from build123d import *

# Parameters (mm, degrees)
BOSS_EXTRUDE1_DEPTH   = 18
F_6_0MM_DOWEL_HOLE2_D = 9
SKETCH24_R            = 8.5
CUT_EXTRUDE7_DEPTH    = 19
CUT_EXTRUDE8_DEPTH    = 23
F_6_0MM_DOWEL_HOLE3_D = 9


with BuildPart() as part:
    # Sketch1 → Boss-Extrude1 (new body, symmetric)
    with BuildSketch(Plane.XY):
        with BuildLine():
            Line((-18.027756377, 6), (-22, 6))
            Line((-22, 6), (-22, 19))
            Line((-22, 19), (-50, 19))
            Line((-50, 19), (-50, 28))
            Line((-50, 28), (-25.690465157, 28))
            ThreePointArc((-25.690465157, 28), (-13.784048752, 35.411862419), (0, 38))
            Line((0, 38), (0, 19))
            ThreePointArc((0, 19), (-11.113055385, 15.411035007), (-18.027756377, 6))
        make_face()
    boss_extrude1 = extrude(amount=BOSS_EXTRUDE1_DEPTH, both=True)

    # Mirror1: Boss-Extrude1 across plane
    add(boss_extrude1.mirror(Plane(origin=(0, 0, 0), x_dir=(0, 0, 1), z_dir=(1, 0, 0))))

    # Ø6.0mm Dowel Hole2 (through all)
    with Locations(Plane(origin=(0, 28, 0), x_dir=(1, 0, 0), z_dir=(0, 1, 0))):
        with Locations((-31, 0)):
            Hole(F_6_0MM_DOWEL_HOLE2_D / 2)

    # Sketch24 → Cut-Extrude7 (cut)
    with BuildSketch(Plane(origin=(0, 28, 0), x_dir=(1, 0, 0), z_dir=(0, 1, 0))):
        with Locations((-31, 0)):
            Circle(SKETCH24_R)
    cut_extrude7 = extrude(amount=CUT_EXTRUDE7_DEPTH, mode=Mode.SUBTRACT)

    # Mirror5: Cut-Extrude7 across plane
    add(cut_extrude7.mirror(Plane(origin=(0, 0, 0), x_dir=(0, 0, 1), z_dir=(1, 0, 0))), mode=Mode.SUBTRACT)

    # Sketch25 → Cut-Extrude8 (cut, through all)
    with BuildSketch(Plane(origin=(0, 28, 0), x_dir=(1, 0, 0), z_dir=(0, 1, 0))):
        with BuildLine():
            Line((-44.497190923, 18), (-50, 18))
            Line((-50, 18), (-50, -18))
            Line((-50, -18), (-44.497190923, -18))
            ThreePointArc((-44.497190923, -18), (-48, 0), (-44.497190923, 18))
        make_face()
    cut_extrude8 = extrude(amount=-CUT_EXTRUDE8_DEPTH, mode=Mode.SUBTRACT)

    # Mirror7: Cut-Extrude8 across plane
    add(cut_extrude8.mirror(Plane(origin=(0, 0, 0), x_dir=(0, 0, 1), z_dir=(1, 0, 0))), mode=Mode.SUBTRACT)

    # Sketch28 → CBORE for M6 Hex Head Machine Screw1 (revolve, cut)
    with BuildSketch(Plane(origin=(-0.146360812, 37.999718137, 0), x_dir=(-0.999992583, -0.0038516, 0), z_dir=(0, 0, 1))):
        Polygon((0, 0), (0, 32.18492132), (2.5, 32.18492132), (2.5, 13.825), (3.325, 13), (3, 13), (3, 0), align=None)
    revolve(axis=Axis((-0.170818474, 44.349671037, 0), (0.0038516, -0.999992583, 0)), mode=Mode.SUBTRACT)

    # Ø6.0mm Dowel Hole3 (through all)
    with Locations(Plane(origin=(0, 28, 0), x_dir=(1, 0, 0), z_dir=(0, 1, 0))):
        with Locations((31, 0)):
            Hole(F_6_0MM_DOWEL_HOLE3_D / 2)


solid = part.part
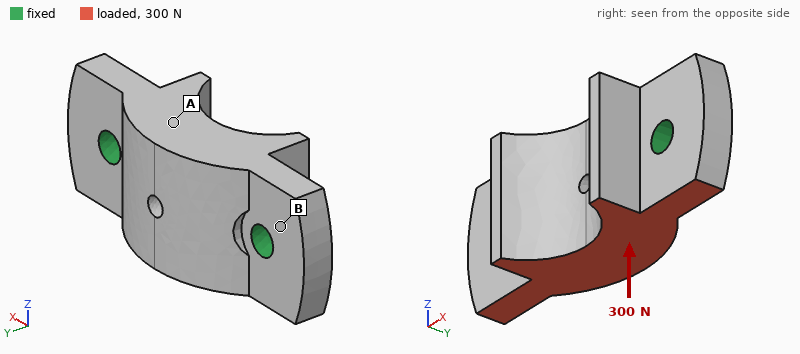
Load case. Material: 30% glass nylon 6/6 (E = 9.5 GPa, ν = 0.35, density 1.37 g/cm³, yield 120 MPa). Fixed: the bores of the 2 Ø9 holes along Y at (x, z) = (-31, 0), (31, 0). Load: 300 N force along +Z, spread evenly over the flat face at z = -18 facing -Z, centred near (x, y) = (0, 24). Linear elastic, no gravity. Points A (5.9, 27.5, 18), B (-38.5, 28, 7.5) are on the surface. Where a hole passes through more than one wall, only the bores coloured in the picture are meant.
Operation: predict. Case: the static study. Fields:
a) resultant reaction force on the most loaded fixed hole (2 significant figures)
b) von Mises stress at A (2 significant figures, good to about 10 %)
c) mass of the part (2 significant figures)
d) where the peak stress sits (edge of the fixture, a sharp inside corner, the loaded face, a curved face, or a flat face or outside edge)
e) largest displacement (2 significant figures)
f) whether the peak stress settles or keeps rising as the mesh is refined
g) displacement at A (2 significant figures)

150 N
0.38 MPa
68 g
edge of the fixture
3.3 µm
keeps rising
2.2 µm
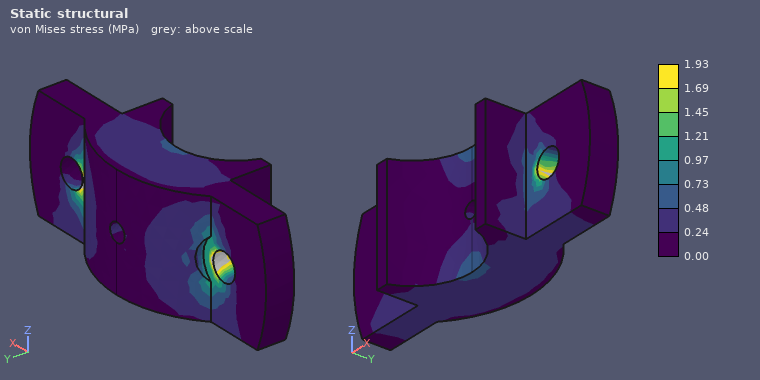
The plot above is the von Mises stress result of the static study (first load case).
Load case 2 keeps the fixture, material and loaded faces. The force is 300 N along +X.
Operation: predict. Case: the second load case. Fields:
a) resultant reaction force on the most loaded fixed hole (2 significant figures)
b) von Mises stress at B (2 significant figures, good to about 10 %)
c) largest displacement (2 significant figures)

170 N
0.27 MPa
3.6 µm
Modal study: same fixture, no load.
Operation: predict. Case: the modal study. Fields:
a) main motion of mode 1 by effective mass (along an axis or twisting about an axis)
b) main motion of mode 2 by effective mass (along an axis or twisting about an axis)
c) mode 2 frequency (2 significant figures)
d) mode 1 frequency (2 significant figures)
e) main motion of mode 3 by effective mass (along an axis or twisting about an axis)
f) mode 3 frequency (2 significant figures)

twisting about X
along Y
6000 Hz
4700 Hz
along Z
7600 Hz
